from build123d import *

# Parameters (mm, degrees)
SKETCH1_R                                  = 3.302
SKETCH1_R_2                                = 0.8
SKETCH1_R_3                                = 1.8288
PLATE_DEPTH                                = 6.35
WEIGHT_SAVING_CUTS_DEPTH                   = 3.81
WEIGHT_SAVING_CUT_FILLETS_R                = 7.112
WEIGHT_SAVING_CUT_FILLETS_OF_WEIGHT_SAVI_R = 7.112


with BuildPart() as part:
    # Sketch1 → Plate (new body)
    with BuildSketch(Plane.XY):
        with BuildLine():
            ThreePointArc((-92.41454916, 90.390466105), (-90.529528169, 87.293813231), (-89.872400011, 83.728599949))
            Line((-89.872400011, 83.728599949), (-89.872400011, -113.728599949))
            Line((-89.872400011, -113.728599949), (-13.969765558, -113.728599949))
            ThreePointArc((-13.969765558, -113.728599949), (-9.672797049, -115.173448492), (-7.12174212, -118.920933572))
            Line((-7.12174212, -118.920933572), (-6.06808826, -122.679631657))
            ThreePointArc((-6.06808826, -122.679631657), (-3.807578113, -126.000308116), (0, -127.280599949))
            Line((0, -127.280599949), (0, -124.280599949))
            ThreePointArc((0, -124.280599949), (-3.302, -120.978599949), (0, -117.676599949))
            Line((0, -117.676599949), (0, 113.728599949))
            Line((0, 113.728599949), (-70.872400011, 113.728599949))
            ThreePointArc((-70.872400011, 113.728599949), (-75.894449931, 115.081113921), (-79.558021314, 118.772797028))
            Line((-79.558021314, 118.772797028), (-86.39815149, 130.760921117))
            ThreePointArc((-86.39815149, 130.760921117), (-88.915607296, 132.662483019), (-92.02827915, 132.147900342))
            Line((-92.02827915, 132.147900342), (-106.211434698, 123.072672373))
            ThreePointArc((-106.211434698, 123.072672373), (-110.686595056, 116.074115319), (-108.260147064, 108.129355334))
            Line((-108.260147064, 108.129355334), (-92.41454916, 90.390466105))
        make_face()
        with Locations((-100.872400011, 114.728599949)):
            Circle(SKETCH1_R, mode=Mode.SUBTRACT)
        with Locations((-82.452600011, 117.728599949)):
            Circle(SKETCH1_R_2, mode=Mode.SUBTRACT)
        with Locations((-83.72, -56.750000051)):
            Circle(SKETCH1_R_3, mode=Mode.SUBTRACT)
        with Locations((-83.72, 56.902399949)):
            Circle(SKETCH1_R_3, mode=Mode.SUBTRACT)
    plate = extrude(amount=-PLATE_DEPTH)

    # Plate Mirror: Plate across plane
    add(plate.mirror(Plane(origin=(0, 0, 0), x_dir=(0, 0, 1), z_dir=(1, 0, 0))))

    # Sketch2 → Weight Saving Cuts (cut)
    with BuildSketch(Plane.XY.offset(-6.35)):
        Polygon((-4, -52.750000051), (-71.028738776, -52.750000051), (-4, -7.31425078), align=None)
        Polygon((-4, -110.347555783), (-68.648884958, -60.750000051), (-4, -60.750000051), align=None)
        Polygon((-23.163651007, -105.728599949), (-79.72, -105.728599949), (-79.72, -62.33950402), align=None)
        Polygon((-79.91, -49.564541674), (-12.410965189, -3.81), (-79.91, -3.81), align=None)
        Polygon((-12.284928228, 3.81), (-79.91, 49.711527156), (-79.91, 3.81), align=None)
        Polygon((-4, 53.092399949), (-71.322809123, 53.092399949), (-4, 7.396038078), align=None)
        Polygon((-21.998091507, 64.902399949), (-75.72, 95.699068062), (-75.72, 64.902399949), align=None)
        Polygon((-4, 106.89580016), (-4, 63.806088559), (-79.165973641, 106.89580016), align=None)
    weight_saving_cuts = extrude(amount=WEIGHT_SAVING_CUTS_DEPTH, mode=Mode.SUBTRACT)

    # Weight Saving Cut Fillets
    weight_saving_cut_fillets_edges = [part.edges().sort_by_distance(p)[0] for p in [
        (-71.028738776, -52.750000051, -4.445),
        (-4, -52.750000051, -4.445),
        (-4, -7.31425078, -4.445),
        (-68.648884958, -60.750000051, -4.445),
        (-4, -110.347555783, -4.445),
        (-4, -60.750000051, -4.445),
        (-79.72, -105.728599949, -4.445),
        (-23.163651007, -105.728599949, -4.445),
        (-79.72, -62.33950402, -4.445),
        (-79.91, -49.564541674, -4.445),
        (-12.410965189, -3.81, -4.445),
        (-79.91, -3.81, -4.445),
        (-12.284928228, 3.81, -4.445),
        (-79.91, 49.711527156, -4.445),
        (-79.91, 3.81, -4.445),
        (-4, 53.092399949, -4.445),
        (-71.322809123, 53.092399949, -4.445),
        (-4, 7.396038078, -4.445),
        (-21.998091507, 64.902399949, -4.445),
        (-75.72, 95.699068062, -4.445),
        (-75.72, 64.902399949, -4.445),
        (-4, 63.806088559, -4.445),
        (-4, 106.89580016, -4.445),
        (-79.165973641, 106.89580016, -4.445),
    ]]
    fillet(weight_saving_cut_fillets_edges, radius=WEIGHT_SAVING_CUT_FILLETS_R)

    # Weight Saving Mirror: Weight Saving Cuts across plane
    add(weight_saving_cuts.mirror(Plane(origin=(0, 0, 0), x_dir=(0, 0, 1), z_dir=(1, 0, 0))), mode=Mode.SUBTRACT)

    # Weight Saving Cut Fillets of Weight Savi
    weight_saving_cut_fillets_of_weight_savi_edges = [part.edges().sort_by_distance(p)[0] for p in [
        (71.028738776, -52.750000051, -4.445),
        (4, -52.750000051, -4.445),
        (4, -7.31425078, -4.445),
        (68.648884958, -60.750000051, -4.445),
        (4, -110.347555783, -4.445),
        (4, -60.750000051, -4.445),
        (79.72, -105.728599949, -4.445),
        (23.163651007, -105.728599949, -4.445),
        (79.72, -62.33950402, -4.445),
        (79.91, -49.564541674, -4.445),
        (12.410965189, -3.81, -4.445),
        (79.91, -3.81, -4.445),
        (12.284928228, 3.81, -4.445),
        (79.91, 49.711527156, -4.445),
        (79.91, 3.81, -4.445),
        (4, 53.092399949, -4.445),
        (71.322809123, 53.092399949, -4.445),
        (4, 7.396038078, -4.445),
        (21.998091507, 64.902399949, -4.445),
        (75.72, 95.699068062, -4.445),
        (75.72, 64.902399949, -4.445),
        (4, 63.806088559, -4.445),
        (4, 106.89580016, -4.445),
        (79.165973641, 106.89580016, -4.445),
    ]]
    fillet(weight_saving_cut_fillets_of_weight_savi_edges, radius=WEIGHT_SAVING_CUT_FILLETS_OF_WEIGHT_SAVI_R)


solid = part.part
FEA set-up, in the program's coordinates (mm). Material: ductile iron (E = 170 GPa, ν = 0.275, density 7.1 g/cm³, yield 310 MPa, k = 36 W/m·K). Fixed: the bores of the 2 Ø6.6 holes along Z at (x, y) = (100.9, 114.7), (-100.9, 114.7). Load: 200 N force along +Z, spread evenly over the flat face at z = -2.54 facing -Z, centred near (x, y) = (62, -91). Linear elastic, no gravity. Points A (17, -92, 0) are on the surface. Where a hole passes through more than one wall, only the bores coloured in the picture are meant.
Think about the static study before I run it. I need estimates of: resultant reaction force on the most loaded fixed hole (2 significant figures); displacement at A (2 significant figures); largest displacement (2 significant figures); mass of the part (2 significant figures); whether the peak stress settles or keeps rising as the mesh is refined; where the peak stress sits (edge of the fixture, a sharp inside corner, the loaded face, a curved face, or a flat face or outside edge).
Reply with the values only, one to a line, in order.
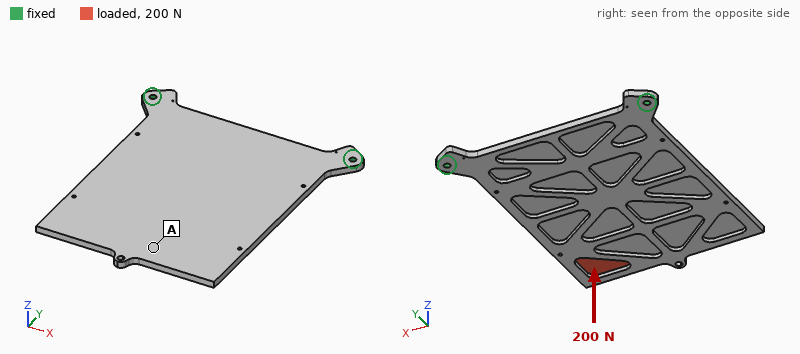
380 N
2.7 mm
3.3 mm
1.4 kg
keeps rising
edge of the fixture
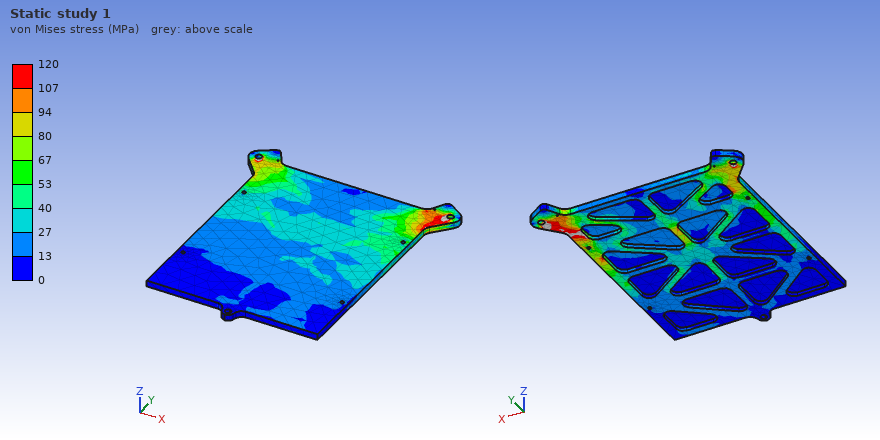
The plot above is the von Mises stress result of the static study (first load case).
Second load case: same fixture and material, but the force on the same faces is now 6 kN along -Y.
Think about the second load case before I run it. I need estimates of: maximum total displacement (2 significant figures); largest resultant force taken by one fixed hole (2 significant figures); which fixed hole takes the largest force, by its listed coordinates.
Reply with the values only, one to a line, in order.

98 µm
5.3 kN
(100.9, 114.7)
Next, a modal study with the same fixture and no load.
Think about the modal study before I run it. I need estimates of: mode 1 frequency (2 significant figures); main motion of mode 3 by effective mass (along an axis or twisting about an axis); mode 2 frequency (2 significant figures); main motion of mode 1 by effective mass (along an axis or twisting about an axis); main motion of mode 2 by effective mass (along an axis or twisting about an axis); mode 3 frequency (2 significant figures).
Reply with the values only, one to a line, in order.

65 Hz
along Z
240 Hz
along Z
twisting about Y
400 Hz
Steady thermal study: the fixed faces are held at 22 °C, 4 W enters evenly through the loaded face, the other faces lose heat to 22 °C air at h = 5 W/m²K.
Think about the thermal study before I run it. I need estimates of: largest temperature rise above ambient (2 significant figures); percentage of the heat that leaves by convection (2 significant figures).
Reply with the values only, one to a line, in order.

25 K
83 %
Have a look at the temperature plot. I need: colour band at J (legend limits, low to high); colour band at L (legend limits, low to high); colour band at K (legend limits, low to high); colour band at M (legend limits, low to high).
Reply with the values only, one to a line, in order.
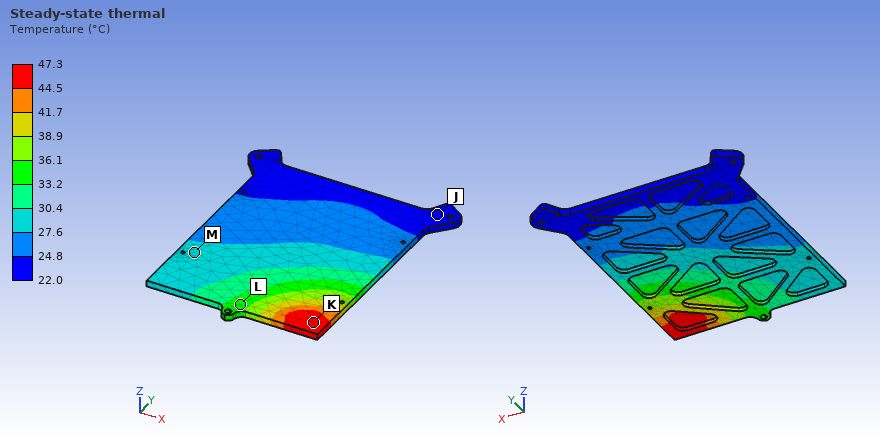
22.0 to 24.8 °C
33.2 to 36.1 °C
44.5 to 47.3 °C
27.6 to 30.4 °C
